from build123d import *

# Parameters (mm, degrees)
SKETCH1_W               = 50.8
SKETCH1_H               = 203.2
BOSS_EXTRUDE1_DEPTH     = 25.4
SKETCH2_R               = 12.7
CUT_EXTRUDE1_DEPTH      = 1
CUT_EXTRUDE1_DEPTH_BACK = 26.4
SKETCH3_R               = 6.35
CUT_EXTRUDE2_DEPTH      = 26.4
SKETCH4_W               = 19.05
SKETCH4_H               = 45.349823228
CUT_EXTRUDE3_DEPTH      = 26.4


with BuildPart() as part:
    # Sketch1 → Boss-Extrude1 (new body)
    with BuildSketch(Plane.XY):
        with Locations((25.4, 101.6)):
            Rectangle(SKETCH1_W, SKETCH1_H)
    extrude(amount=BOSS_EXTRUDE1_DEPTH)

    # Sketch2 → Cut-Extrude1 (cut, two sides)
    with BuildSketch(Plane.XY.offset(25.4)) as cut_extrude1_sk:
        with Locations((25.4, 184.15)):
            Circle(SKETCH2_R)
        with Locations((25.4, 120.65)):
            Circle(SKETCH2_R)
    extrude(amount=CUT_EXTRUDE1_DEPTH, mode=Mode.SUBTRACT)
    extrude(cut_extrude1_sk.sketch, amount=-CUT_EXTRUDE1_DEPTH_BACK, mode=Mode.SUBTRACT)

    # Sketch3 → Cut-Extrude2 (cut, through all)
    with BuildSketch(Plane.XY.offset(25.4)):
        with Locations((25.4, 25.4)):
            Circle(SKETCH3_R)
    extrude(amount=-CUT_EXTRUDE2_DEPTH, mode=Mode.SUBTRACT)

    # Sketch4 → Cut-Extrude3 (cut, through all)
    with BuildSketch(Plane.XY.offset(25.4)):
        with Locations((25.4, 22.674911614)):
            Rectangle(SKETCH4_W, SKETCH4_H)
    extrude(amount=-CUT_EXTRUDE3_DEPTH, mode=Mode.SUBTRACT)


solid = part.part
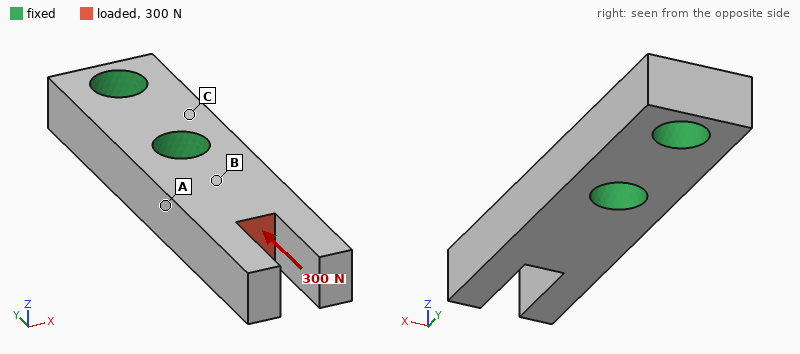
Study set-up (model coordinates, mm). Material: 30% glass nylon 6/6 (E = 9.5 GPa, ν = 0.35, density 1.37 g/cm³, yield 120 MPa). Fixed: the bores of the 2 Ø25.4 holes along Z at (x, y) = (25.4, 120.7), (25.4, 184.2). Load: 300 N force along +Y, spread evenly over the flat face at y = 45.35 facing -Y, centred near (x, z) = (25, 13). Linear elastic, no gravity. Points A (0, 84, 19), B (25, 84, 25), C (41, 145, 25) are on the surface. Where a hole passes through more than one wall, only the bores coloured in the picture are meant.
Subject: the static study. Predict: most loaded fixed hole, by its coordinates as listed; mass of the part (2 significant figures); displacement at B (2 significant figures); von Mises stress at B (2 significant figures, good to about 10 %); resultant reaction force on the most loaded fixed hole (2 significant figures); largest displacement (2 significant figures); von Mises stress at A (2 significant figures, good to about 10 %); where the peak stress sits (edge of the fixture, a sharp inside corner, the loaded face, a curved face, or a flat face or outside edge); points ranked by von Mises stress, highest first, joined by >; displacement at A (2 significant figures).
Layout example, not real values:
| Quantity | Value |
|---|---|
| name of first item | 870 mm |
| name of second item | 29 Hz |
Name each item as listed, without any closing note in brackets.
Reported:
| Quantity | Value |
|---|---|
| most loaded fixed hole, by its coordinates as listed | (25.4, 120.7) |
| mass of the part | 290 g |
| displacement at B | 0.78 µm |
| von Mises stress at B | 0.31 MPa |
| resultant reaction force on the most loaded fixed hole | 290 N |
| largest displacement | 3.4 µm |
| von Mises stress at A | 0.18 MPa |
| where the peak stress sits | a flat face or outside edge |
| points ranked by von Mises stress, highest first, joined by > | B > A > C |
| displacement at A | 0.84 µm |
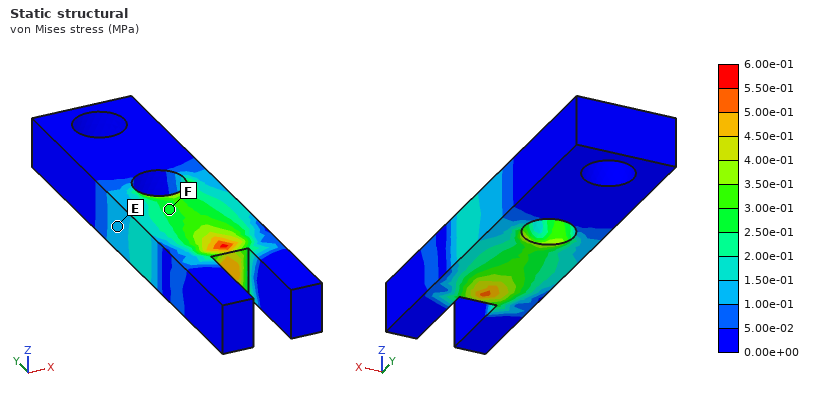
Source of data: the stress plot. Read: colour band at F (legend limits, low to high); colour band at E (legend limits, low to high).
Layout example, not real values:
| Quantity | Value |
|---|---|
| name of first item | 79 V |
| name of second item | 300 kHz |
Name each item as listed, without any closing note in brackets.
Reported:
| Quantity | Value |
|---|---|
| colour band at F | 2.50e-01 to 3.00e-01 MPa |
| colour band at E | 1.00e-01 to 1.50e-01 MPa |
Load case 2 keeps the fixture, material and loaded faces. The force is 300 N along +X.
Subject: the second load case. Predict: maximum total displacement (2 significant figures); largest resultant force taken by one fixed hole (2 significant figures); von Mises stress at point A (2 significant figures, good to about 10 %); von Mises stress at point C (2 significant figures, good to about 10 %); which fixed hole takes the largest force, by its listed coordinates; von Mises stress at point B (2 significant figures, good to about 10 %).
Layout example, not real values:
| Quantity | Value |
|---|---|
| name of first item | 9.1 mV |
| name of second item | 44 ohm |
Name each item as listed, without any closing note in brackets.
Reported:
| Quantity | Value |
|---|---|
| maximum total displacement | 40 µm |
| largest resultant force taken by one fixed hole | 360 N |
| von Mises stress at point A | 1.1 MPa |
| von Mises stress at point C | 0.18 MPa |
| which fixed hole takes the largest force, by its listed coordinates | (25.4, 120.7) |
| von Mises stress at point B | 0.63 MPa |
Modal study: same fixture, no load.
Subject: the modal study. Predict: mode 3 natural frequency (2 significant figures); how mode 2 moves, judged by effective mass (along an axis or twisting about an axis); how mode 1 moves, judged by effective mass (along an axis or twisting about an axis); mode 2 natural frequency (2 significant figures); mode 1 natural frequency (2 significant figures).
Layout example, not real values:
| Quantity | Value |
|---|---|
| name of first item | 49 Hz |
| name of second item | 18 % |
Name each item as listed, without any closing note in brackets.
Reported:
| Quantity | Value |
|---|---|
| mode 3 natural frequency | 2100 Hz |
| how mode 2 moves, judged by effective mass | along X |
| how mode 1 moves, judged by effective mass | along Z |
| mode 2 natural frequency | 1400 Hz |
| mode 1 natural frequency | 1000 Hz |
